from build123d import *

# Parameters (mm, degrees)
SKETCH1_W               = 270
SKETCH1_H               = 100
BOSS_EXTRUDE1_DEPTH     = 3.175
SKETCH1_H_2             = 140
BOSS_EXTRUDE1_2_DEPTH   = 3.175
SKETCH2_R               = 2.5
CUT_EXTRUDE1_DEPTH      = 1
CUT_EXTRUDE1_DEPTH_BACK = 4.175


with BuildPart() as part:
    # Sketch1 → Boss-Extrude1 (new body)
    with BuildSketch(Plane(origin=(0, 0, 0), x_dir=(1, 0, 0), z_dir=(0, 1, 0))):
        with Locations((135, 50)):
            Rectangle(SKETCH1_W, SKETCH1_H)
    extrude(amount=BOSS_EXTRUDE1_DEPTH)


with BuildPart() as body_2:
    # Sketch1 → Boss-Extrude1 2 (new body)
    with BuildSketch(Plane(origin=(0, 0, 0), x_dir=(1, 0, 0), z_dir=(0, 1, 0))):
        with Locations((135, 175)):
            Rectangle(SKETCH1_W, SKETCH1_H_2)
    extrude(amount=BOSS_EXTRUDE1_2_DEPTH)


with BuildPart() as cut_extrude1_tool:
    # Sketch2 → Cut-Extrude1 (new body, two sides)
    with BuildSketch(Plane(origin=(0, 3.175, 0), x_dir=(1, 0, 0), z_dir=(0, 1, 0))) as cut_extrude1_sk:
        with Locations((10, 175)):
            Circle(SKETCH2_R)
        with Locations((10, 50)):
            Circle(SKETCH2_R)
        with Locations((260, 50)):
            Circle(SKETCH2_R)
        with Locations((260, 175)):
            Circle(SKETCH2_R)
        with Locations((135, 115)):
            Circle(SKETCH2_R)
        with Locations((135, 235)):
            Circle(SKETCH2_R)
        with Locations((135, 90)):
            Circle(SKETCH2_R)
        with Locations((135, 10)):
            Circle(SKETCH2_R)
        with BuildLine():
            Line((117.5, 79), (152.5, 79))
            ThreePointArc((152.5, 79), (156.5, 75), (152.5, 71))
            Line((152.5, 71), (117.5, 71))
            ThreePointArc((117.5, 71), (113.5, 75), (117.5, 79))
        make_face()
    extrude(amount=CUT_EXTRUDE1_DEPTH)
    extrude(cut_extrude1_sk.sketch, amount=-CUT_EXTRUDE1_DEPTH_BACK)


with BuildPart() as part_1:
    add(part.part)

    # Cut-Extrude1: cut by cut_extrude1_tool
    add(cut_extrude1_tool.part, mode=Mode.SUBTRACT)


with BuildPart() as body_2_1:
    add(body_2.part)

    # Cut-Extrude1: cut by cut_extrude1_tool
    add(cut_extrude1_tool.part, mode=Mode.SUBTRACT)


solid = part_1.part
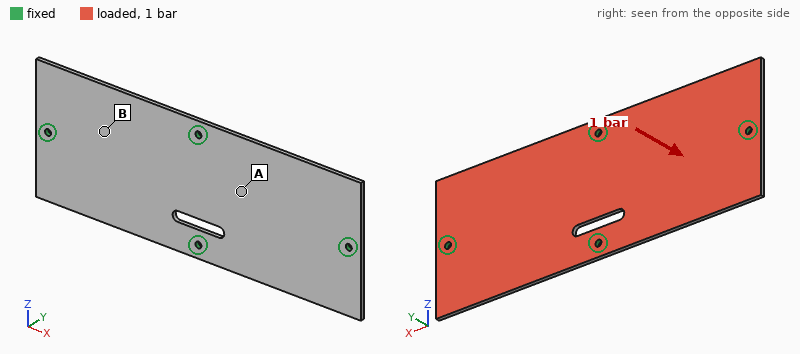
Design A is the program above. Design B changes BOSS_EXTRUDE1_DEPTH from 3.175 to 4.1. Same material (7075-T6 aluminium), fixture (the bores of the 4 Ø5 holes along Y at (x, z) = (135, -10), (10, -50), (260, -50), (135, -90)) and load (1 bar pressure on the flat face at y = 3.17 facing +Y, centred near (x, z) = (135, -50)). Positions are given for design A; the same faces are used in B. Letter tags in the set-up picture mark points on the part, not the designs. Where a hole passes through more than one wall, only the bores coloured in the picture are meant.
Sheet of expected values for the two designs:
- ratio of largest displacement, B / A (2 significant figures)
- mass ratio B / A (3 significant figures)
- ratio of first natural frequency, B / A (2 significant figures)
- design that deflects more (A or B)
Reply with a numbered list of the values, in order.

1. 0.47
2. 1.29
3. 1.3
4. A
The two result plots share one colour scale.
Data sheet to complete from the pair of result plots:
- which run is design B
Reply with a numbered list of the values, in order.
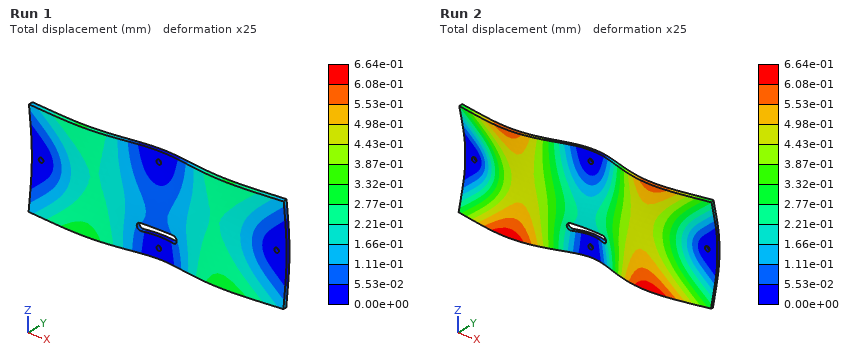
1. Run 1
